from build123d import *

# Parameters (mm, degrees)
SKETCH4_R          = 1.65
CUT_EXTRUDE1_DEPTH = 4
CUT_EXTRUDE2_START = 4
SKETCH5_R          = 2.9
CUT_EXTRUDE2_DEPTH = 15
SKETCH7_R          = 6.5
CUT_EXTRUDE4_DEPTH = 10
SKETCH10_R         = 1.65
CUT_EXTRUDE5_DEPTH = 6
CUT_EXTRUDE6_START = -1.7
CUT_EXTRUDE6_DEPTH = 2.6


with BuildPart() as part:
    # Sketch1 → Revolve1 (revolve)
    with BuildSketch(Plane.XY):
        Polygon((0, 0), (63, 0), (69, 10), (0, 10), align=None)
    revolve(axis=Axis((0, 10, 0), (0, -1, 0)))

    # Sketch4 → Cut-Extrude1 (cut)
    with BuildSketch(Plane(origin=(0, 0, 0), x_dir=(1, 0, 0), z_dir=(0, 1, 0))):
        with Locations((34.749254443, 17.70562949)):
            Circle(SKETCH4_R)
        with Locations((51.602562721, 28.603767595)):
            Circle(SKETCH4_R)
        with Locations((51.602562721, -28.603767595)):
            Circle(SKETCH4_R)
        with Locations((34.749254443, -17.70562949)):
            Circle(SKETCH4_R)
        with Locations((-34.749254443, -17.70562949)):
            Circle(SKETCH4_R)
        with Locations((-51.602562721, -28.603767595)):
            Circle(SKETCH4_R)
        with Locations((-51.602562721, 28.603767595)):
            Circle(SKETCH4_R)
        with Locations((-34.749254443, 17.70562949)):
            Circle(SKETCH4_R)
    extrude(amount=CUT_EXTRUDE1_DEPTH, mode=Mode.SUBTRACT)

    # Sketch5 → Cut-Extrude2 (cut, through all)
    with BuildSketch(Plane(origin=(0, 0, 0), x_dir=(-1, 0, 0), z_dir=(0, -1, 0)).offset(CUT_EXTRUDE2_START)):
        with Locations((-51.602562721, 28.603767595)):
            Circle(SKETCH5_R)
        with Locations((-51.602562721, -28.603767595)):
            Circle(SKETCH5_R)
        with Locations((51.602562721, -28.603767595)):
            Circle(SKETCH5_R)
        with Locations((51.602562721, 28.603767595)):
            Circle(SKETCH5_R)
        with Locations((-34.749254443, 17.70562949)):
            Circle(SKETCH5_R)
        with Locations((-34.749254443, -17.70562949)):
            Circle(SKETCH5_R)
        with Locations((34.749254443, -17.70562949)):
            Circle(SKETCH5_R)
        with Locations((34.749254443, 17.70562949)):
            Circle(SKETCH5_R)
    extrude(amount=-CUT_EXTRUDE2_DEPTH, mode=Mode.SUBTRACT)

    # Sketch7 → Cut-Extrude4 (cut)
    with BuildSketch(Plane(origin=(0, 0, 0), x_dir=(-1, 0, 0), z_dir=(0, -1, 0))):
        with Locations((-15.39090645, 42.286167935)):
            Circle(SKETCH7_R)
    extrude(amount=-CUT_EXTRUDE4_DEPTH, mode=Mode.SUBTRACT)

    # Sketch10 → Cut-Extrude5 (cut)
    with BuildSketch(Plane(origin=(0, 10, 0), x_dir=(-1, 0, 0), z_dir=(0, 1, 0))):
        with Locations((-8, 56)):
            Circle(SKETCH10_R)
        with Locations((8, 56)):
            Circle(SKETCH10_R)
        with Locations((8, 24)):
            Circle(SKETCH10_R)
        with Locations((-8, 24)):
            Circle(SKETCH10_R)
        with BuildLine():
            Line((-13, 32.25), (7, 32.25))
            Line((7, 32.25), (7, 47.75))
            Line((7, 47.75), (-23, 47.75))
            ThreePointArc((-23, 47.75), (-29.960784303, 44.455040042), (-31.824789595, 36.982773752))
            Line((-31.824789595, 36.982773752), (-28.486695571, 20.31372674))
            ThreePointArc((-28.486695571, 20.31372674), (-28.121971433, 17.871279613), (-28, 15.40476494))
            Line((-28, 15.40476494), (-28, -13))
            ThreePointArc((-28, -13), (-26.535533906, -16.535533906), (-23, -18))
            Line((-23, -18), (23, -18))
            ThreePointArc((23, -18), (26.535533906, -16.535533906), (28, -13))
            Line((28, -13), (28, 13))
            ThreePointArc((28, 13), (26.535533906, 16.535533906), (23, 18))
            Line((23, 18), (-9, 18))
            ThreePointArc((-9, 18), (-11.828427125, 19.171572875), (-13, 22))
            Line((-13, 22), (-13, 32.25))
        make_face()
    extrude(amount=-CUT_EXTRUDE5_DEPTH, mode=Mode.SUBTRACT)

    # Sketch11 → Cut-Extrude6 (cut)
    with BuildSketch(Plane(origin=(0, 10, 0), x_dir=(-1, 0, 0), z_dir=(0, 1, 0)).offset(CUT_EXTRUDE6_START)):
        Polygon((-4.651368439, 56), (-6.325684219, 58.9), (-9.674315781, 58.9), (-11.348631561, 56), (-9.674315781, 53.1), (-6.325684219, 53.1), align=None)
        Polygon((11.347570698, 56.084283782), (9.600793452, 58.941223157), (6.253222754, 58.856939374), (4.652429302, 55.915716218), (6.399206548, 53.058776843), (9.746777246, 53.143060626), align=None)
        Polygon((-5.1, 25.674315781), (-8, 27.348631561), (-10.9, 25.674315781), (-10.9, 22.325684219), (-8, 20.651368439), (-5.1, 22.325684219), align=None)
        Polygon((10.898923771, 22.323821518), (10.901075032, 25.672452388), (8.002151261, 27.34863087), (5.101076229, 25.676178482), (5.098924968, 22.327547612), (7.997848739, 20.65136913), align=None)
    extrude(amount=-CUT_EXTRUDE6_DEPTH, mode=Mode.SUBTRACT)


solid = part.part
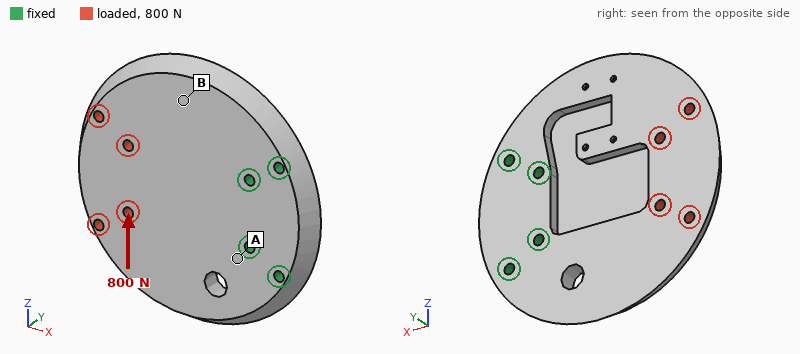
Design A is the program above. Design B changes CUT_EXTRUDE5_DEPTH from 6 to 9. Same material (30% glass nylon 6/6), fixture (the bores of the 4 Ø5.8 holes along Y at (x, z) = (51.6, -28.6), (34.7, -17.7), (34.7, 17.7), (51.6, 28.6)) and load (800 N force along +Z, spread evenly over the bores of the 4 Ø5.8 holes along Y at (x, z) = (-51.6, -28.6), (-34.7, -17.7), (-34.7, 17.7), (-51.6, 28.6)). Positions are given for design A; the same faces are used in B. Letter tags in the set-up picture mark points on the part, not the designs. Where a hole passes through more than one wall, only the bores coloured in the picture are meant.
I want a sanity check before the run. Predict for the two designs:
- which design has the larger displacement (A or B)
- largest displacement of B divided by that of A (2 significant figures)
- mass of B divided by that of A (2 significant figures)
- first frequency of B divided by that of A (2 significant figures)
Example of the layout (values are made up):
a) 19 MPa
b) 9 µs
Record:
a) B
b) 1.4
c) 0.93
d) 0.94
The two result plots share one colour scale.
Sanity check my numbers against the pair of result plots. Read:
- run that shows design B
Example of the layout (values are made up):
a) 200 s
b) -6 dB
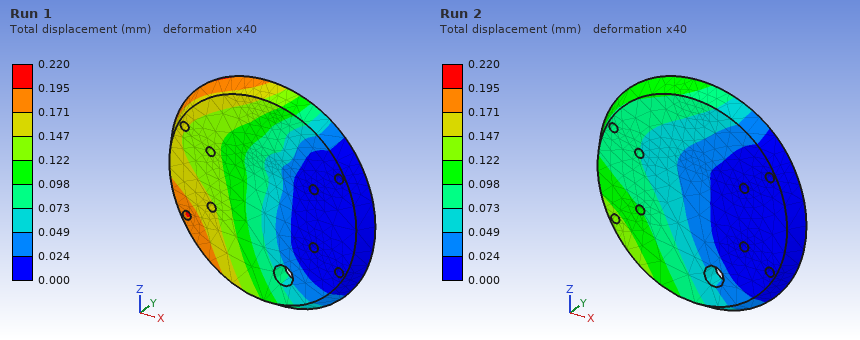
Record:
a) Run 1
